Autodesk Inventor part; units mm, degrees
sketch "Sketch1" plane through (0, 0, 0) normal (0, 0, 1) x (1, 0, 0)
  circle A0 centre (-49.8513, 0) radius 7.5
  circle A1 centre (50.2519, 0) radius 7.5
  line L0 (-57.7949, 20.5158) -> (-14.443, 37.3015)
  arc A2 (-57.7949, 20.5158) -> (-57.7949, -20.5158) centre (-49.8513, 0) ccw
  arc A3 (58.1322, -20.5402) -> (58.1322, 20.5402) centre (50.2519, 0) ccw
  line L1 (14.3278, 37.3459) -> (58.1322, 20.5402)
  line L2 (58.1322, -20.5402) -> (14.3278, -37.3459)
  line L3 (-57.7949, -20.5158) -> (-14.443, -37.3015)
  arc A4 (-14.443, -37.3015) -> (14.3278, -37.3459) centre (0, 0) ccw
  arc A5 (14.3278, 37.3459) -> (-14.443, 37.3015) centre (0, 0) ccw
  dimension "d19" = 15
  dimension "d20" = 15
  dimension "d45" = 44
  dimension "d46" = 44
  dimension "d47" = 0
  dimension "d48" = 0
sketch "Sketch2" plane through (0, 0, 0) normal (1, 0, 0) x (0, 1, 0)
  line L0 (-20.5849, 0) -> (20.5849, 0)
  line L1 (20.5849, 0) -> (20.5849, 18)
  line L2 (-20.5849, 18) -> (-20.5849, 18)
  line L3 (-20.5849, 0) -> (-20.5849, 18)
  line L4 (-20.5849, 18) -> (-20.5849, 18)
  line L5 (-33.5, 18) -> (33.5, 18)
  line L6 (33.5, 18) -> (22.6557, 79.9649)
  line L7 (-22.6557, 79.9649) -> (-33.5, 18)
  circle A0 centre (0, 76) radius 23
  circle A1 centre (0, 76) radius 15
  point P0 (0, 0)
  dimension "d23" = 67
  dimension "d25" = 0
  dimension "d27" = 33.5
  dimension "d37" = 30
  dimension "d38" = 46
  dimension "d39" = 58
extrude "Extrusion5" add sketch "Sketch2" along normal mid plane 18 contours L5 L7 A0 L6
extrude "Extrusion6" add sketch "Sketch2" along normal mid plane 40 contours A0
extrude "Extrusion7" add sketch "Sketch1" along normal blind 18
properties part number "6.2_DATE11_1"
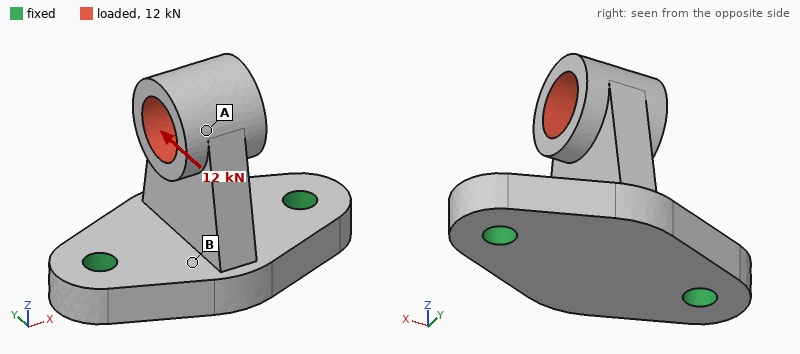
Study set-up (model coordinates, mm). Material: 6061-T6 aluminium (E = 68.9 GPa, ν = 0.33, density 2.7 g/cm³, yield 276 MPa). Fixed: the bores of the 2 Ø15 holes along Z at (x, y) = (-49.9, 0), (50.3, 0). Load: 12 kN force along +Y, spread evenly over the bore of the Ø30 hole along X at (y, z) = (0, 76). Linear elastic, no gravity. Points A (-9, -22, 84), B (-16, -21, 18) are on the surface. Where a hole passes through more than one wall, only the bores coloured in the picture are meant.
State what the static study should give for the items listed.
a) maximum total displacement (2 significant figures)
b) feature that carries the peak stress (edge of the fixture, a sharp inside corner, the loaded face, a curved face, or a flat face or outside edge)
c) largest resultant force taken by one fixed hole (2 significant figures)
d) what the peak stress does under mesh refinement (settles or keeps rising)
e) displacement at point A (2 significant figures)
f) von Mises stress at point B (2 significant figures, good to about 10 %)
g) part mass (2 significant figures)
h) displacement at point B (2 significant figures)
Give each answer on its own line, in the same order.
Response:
0.59 mm
edge of the fixture
6.0 kN
keeps rising
0.51 mm
62 MPa
600 g
0.11 mm
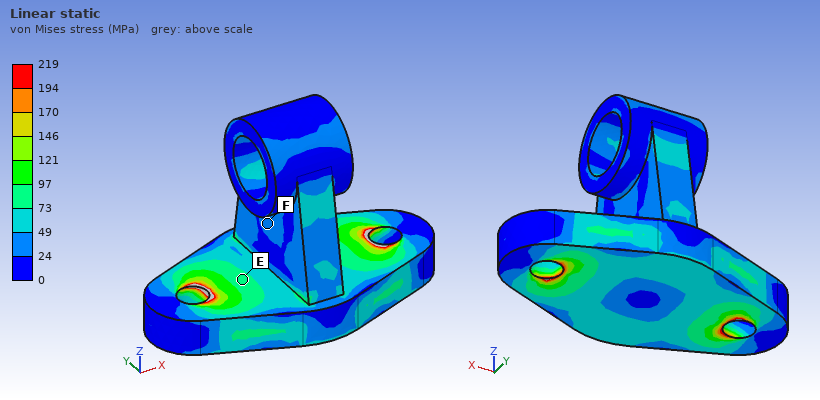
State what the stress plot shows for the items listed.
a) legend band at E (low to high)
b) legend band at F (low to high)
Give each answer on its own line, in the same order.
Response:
73 to 97 MPa
24 to 49 MPa
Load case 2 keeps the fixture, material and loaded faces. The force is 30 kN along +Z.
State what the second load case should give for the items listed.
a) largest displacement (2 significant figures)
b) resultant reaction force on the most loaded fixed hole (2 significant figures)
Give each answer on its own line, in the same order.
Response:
0.14 mm
15 kN
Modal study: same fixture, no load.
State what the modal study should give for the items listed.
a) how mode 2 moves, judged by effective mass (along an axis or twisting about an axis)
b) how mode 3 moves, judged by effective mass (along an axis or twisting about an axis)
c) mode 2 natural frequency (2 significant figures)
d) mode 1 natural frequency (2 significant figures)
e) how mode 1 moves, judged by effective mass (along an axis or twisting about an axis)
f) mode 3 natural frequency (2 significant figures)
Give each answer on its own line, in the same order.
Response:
along Y
along Z
2100 Hz
1900 Hz
along X
4700 Hz
